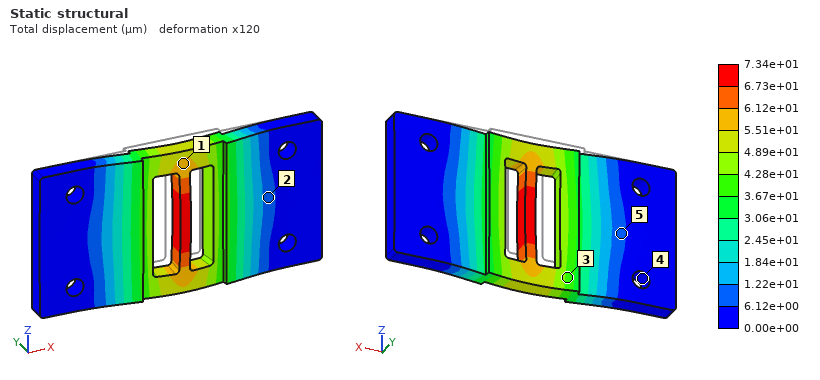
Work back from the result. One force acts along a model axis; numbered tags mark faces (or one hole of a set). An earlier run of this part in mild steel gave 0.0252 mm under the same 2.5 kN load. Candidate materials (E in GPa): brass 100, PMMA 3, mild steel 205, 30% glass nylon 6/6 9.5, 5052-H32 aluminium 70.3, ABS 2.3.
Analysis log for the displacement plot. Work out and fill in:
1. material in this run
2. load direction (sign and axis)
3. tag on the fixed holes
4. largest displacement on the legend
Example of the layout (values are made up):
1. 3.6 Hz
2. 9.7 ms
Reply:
1. 5052-H32 aluminium
2. -Y
3. 4
4. 7.34e+01 µm
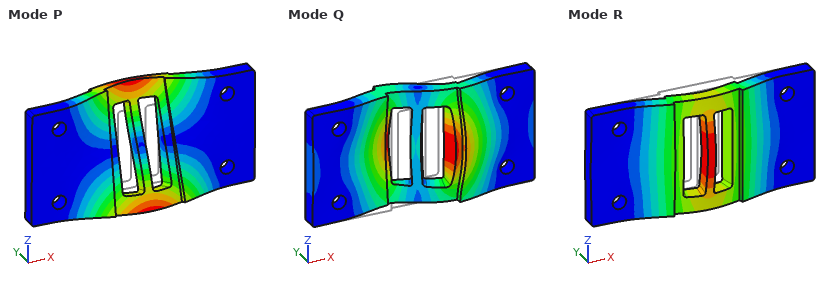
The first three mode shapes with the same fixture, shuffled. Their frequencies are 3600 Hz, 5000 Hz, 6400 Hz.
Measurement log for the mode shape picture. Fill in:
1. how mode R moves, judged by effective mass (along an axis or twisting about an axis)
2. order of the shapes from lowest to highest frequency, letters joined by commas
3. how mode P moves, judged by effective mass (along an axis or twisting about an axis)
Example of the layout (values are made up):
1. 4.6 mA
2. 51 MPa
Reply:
1. along Y
2. R, P, Q
3. twisting about X
